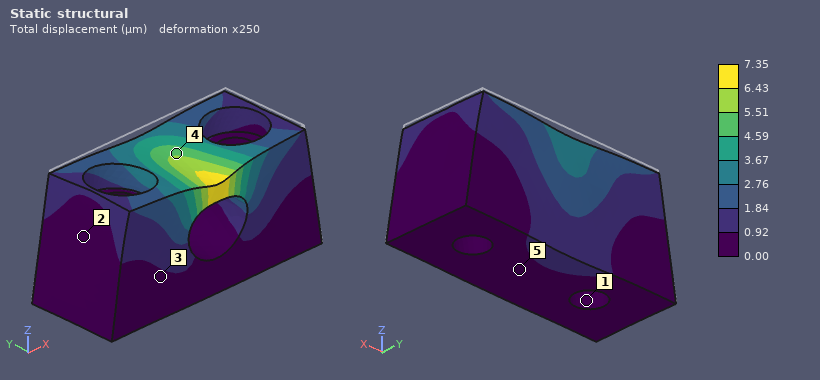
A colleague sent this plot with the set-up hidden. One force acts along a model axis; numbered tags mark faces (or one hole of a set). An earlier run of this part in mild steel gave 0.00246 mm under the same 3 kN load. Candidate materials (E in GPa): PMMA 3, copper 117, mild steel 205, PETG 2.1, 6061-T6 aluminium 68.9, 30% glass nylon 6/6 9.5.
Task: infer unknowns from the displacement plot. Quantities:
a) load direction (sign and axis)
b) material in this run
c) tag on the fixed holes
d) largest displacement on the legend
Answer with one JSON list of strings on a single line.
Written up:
["-Z", "6061-T6 aluminium", "1", "7.35 µm"]
